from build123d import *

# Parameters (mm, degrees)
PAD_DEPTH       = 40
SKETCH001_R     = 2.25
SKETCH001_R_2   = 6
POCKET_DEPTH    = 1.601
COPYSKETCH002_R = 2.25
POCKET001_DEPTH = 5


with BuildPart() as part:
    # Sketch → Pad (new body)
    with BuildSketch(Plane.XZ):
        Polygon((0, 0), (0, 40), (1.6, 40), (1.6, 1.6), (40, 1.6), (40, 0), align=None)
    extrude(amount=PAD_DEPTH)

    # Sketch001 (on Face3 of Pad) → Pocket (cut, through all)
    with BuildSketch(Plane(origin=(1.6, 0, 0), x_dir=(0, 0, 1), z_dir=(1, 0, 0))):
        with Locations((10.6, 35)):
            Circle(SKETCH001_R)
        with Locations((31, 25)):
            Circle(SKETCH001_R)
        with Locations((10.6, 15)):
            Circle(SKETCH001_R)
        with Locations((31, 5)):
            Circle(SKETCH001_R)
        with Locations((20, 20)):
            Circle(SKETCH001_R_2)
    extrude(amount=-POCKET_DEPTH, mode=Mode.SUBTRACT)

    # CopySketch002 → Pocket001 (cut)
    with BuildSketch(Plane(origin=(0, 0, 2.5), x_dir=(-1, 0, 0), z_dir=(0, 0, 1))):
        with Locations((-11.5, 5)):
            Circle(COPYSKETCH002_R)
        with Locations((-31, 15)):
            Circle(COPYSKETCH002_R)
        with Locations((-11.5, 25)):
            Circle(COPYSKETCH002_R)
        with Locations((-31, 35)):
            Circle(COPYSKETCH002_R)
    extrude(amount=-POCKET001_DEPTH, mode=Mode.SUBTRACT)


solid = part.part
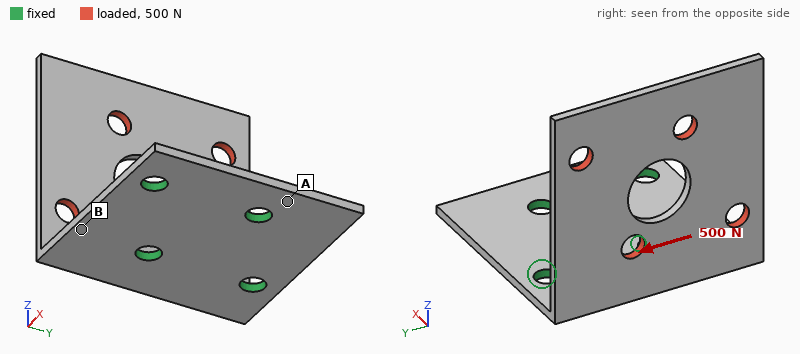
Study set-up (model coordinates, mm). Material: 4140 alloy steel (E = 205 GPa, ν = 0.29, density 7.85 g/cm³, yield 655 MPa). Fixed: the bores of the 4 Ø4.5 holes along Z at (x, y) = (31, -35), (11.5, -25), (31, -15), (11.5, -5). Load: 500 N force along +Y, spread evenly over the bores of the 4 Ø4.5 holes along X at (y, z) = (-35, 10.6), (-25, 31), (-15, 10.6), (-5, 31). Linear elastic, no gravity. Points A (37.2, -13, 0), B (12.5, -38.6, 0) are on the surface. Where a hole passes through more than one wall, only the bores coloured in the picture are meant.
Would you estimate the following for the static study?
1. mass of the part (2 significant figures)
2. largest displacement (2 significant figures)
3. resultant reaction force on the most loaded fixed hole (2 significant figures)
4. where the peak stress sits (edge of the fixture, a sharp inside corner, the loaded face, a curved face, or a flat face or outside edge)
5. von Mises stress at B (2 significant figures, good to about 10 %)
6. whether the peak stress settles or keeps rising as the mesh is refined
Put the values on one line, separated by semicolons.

36 g; 0.30 mm; 540 N; edge of the fixture; 120 MPa; keeps rising
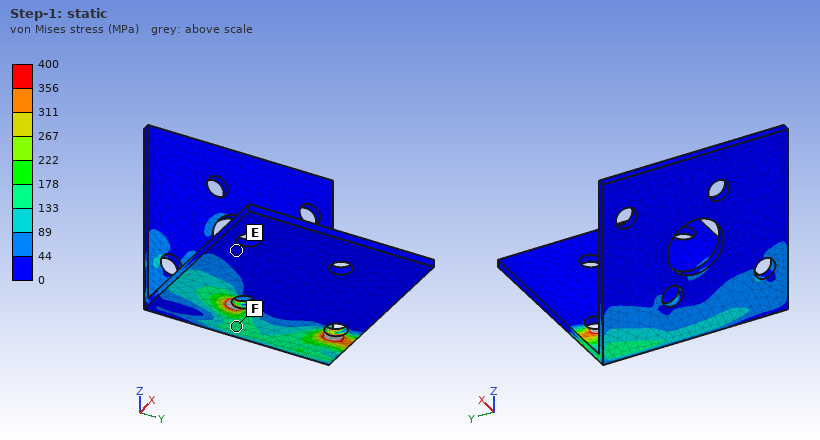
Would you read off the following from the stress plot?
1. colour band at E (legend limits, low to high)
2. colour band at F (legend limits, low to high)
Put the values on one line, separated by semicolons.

0 to 44 MPa; 133 to 178 MPa
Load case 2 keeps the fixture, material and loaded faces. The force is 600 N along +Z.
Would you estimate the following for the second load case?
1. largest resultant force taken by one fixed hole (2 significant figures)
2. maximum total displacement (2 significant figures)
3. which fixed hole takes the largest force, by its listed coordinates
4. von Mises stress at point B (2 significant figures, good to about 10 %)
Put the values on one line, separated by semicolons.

460 N; 0.43 mm; (11.5, -25); 110 MPa
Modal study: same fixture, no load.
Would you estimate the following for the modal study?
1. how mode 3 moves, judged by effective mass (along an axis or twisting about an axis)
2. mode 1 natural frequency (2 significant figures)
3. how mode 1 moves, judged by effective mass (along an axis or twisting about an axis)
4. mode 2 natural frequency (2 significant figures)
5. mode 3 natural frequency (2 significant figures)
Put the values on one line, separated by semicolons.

along Y; 620 Hz; along X; 1600 Hz; 2200 Hz
